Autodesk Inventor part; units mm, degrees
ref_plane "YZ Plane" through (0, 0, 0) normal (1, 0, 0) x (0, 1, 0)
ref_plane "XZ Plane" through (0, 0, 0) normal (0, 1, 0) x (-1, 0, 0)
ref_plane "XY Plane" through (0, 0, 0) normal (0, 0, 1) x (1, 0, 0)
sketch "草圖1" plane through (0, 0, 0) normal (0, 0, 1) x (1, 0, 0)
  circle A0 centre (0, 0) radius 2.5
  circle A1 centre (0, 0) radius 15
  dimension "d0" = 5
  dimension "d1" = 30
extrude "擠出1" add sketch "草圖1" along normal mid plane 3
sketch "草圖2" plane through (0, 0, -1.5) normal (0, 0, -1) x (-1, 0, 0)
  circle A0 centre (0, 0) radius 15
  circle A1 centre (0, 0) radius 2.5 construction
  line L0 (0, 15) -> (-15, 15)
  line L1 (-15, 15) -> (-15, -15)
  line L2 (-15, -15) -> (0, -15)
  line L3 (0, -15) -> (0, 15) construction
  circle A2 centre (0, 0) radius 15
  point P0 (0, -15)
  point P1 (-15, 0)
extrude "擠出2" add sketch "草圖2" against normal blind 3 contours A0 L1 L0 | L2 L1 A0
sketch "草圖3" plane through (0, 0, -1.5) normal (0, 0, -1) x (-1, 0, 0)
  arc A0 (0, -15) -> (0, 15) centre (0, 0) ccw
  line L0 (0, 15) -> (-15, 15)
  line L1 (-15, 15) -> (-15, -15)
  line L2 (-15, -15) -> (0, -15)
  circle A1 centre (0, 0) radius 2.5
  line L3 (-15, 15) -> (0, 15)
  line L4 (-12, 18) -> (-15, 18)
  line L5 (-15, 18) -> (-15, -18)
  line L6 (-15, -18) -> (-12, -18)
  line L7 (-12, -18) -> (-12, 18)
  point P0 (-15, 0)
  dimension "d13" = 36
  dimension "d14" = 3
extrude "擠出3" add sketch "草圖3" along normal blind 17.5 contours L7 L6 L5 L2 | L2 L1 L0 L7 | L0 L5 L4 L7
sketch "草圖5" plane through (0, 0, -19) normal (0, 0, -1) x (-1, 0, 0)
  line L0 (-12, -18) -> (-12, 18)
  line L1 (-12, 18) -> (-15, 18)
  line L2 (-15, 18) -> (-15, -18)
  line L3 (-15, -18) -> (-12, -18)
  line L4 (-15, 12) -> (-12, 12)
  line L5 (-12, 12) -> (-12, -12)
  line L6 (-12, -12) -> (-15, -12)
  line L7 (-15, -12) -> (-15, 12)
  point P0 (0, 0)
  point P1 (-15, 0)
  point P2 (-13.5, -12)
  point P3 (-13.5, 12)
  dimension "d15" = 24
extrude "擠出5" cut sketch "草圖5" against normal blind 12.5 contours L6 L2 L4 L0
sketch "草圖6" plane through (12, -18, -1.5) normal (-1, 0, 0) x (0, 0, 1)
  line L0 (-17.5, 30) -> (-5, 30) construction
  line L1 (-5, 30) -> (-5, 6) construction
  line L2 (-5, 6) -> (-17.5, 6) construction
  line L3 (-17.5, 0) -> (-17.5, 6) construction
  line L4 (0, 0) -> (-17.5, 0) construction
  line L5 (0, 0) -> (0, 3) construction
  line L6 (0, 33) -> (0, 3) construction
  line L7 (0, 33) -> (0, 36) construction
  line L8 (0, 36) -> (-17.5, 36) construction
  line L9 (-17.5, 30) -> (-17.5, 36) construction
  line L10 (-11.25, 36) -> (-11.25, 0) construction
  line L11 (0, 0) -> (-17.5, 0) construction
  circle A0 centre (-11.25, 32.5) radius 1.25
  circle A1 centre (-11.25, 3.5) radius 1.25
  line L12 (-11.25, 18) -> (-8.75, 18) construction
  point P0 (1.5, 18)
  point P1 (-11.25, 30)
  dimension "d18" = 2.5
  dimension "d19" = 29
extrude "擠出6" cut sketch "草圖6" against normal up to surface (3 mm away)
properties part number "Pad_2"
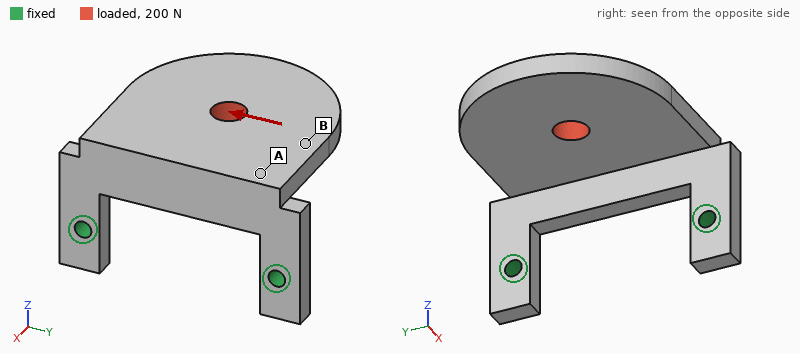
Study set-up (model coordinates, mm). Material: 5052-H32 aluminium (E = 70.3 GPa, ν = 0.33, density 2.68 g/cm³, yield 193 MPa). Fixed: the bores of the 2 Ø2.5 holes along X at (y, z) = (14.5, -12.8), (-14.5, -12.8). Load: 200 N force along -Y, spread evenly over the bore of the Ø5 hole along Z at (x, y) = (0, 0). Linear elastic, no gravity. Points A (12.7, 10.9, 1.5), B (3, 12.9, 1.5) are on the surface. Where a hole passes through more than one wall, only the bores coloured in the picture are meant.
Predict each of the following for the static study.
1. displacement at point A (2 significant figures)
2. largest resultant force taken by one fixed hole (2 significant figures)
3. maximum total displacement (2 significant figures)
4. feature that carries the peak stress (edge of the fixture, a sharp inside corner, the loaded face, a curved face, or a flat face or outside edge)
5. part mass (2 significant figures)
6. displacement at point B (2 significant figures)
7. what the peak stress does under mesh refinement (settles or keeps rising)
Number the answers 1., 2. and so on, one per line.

1. 20 µm
2. 140 N
3. 54 µm
4. edge of the fixture
5. 8.9 g
6. 32 µm
7. keeps rising
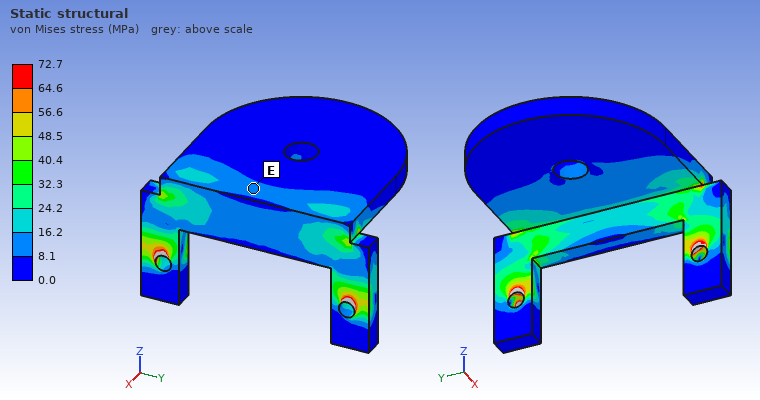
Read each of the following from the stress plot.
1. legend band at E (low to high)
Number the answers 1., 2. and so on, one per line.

1. 8.1 to 16.2 MPa
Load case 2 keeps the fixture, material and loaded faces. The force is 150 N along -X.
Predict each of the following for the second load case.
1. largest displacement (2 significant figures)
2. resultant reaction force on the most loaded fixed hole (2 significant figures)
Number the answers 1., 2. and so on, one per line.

1. 0.17 mm
2. 75 N
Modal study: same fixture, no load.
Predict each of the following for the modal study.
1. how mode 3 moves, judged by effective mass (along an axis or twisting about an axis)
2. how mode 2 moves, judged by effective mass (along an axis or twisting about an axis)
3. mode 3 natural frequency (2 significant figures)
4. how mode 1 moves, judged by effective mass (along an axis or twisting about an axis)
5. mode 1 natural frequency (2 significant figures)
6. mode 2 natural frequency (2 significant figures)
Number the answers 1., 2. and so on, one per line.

1. along X
2. along Y
3. 5600 Hz
4. along Z
5. 1500 Hz
6. 4400 Hz
